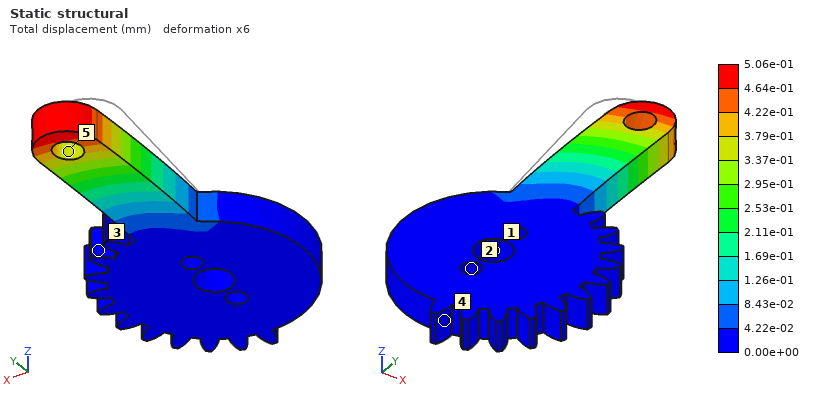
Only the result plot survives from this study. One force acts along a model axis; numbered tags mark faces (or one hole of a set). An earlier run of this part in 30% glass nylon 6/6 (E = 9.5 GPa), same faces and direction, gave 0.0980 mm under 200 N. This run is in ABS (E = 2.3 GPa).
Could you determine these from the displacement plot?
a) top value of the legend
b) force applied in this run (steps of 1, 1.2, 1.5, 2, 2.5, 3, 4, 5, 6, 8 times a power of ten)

5.06e-01 mm
250 N
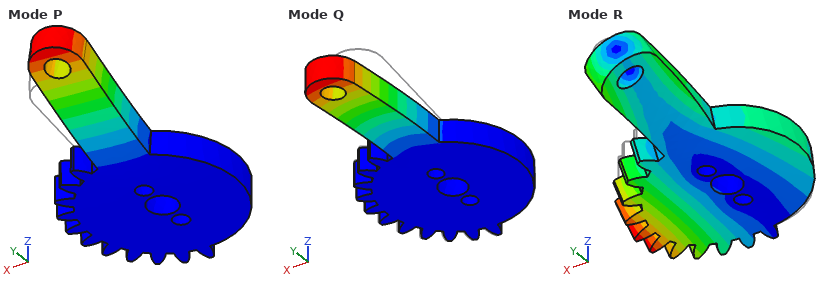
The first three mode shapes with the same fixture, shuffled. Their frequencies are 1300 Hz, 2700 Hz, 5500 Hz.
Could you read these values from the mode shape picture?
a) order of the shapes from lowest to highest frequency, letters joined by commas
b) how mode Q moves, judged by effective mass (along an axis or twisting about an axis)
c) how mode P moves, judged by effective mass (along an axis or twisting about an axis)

P, Q, R
along X
along Z
